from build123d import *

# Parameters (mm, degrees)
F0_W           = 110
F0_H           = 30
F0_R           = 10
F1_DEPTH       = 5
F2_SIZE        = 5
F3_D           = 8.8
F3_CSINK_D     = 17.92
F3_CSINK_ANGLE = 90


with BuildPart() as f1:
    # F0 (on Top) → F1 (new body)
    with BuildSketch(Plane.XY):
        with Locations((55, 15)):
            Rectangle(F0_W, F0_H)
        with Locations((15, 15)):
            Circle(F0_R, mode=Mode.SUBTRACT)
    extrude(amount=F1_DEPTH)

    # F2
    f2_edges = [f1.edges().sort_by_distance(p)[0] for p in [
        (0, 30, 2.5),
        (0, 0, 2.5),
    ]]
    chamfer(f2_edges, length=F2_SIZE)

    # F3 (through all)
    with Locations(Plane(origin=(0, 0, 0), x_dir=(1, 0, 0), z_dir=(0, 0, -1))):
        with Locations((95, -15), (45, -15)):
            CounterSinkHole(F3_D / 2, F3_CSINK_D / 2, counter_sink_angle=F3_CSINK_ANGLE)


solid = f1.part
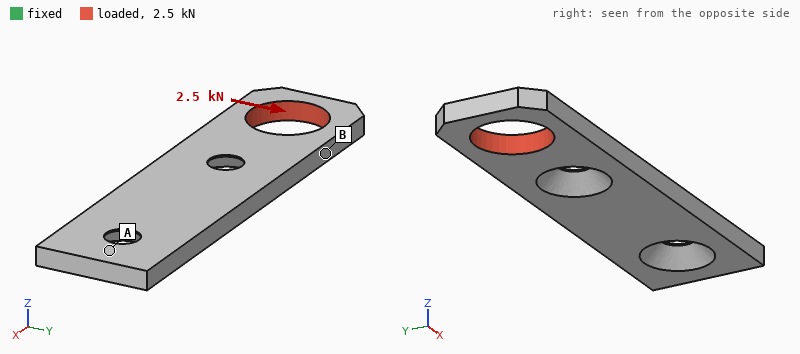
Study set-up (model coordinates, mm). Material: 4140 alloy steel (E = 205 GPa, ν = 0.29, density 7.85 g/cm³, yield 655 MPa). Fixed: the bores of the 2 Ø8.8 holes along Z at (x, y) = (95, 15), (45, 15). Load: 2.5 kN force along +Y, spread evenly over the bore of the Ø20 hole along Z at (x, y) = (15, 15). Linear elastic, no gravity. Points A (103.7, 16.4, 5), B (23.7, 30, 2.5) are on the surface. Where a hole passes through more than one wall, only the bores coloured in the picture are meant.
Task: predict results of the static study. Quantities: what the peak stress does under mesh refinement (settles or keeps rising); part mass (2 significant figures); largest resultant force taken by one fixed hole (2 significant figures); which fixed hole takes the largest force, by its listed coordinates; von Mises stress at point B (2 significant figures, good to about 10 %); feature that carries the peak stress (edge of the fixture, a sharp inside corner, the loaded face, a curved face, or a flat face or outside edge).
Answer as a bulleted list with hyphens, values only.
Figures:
- keeps rising
- 110 g
- 3.6 kN
- (45, 15)
- 120 MPa
- edge of the fixture
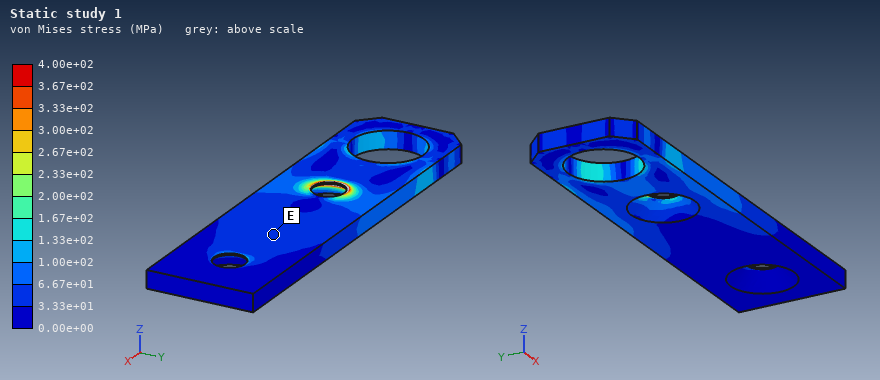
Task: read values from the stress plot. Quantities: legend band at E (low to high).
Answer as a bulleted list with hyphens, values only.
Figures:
- 3.33e+01 to 6.67e+01 MPa
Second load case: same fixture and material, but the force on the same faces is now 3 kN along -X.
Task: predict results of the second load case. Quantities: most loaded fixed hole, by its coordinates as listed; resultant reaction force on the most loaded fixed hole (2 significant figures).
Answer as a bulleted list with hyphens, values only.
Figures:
- (45, 15)
- 2.0 kN
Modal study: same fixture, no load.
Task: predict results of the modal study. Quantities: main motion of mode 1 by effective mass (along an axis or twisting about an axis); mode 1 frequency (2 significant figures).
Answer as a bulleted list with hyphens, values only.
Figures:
- along Z
- 1900 Hz
